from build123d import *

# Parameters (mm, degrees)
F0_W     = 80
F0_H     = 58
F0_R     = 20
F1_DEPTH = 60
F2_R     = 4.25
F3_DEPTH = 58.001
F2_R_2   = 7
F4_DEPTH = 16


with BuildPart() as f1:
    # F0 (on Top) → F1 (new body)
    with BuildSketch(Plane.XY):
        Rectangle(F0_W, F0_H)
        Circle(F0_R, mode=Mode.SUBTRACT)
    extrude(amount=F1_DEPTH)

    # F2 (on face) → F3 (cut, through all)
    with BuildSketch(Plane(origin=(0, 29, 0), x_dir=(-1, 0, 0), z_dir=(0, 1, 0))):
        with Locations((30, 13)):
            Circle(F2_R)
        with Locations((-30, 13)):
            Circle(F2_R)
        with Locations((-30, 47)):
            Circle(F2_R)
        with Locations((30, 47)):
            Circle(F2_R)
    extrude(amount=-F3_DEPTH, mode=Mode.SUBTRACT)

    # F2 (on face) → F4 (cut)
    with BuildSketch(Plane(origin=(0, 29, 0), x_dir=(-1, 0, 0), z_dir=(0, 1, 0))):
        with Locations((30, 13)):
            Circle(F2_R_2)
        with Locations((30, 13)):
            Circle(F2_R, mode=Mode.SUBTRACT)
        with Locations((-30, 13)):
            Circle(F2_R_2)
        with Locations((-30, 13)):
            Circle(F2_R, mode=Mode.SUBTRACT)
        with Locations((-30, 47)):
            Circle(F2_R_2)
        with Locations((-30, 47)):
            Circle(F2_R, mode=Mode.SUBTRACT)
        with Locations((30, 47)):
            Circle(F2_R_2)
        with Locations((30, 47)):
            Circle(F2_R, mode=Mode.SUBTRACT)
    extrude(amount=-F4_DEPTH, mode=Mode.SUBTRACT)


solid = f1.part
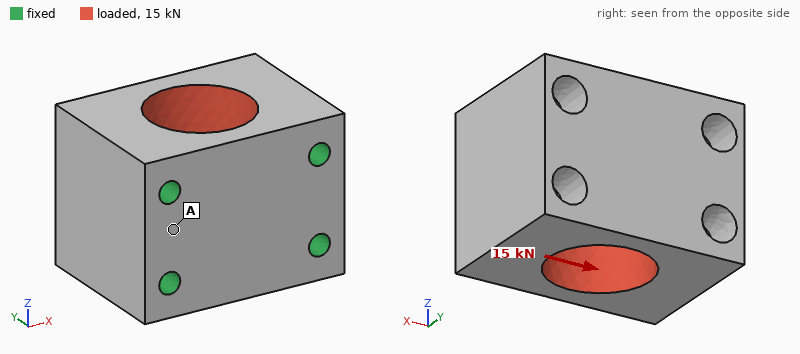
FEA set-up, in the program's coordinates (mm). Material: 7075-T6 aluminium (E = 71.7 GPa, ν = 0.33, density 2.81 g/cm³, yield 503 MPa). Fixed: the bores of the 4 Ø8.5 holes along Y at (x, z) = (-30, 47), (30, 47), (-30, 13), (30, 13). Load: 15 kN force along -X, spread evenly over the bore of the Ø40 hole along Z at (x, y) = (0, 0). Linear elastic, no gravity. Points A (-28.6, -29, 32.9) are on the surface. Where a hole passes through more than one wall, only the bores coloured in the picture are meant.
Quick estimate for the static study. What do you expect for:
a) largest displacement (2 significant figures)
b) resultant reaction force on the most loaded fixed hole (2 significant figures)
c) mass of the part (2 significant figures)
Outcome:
3.2 µm
3.8 kN
520 g
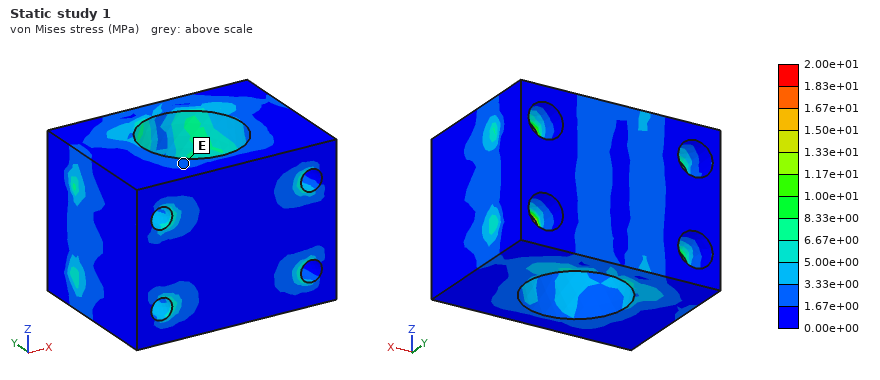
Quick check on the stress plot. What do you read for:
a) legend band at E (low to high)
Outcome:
1.67e+00 to 3.33e+00 MPa
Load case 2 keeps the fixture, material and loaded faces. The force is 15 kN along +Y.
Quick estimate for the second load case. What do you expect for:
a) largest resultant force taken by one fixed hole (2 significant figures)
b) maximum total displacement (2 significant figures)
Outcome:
3.8 kN
4.5 µm
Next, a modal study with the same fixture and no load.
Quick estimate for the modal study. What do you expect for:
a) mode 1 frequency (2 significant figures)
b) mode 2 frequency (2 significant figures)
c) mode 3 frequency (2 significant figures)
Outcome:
18 kHz
18 kHz
22 kHz
